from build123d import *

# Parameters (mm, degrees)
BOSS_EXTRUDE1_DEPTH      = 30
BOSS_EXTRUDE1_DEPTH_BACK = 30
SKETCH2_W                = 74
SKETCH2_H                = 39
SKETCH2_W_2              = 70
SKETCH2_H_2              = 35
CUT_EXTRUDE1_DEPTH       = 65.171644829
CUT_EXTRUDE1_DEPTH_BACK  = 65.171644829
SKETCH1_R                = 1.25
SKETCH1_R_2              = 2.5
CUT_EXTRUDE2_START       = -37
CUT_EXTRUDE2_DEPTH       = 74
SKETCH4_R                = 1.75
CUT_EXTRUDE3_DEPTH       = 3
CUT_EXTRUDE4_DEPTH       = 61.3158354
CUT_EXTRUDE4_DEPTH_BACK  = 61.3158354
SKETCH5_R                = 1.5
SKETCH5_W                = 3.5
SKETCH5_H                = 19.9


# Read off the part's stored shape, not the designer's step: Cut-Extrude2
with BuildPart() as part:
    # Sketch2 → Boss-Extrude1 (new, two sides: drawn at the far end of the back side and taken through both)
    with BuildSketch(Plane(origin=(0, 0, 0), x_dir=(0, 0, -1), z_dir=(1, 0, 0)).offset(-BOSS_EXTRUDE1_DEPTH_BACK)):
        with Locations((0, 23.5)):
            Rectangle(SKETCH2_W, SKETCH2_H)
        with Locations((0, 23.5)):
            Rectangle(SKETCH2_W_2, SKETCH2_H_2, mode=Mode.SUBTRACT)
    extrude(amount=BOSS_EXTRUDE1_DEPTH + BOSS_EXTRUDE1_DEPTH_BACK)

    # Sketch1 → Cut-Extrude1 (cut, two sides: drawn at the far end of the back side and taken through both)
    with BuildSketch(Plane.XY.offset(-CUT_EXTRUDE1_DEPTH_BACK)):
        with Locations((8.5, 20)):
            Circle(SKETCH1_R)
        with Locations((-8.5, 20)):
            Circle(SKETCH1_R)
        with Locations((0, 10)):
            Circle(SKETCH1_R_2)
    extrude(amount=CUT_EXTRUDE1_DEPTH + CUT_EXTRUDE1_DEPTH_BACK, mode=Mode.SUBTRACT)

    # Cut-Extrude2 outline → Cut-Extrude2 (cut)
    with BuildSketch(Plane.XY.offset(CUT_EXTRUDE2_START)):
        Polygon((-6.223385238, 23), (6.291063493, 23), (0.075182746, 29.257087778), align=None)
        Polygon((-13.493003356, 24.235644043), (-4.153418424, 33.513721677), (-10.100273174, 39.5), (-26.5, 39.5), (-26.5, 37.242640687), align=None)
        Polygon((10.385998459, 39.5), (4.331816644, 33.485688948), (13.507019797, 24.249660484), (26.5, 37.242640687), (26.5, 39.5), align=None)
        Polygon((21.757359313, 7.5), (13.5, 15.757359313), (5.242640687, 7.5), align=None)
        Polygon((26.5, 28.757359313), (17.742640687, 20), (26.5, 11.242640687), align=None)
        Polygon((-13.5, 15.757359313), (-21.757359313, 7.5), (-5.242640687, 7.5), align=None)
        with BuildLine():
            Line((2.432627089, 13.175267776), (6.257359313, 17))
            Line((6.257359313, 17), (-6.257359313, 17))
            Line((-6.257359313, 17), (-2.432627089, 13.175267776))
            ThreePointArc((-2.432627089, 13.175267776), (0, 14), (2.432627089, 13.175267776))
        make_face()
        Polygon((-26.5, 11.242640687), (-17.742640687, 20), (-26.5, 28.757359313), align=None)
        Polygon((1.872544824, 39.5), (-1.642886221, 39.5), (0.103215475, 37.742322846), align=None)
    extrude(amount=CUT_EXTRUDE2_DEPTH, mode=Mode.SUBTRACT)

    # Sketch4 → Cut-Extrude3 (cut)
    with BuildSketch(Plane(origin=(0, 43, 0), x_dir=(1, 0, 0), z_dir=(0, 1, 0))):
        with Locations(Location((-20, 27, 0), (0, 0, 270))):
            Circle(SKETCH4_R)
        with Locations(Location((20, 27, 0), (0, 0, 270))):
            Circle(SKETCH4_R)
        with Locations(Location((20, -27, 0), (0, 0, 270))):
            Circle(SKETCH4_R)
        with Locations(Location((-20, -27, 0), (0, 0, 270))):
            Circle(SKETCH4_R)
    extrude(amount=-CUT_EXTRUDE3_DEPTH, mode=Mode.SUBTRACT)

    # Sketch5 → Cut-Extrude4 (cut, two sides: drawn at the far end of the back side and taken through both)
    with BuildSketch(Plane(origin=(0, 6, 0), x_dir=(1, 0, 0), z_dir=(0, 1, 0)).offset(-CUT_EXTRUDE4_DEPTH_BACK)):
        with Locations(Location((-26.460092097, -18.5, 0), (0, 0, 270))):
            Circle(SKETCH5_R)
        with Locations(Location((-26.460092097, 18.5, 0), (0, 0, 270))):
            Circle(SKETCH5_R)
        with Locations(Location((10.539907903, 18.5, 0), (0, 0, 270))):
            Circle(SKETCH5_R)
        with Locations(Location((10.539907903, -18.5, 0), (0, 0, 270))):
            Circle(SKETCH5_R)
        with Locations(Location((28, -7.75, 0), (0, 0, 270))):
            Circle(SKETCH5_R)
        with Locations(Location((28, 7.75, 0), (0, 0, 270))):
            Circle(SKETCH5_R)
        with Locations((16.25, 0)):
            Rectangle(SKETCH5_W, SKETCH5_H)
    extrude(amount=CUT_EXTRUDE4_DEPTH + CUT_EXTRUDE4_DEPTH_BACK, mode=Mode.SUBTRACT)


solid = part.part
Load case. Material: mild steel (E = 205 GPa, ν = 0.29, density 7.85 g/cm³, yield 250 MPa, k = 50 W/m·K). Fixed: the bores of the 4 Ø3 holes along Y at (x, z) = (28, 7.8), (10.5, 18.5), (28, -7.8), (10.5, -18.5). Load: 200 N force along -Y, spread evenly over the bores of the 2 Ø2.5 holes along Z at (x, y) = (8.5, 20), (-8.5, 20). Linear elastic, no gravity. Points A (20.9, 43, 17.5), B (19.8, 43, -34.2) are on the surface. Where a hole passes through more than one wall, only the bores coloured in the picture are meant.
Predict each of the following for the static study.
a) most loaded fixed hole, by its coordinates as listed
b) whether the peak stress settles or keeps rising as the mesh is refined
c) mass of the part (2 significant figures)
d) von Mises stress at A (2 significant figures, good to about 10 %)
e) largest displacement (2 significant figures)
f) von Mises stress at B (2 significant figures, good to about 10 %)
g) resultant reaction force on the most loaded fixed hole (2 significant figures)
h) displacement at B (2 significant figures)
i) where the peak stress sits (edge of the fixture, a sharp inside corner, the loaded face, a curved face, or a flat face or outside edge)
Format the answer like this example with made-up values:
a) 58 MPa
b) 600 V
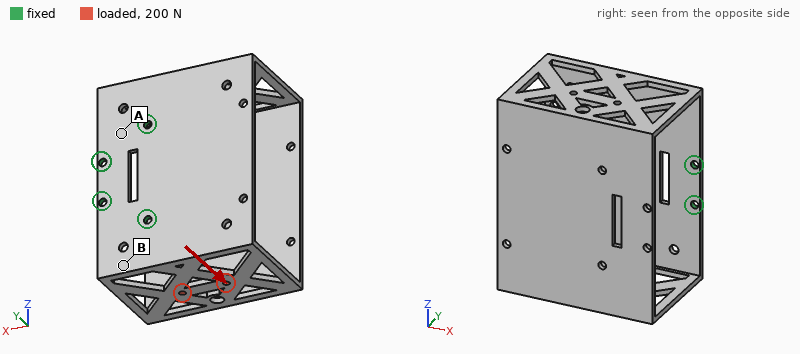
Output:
a) (10.5, -18.5)
b) keeps rising
c) 180 g
d) 18 MPa
e) 0.18 mm
f) 33 MPa
g) 280 N
h) 0.040 mm
i) edge of the fixture
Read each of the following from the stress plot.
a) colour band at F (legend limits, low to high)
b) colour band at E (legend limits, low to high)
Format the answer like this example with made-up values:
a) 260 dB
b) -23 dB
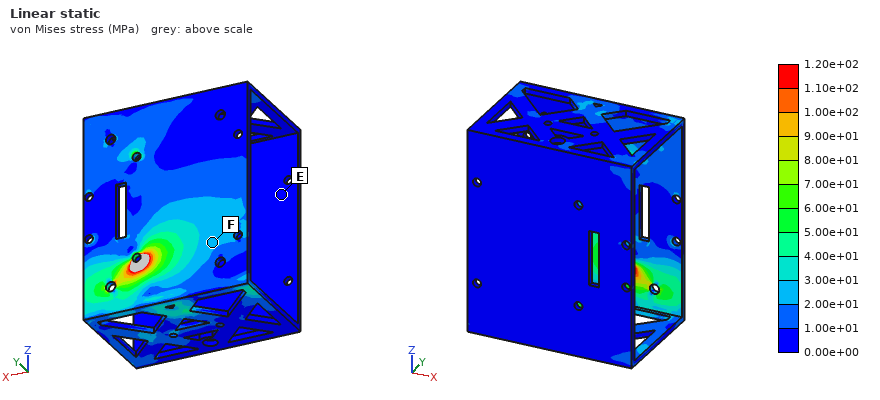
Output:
a) 2.00e+01 to 3.00e+01 MPa
b) 0.00e+00 to 1.00e+01 MPa
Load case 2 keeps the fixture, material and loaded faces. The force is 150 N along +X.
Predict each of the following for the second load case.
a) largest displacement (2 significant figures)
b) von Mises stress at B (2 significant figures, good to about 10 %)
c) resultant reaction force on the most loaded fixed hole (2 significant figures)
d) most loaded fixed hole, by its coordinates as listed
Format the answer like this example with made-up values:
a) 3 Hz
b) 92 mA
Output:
a) 0.20 mm
b) 28 MPa
c) 180 N
d) (10.5, -18.5)
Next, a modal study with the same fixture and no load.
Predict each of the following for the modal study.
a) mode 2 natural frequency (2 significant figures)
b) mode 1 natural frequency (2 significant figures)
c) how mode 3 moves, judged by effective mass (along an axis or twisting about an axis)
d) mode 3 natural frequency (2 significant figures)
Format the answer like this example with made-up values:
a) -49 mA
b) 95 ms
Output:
a) 420 Hz
b) 420 Hz
c) twisting about Y
d) 900 Hz
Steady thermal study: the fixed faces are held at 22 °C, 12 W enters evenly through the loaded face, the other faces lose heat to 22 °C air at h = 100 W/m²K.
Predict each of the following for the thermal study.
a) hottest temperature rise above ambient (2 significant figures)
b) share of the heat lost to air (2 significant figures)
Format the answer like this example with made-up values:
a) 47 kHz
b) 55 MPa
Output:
a) 54 K
b) 94 %
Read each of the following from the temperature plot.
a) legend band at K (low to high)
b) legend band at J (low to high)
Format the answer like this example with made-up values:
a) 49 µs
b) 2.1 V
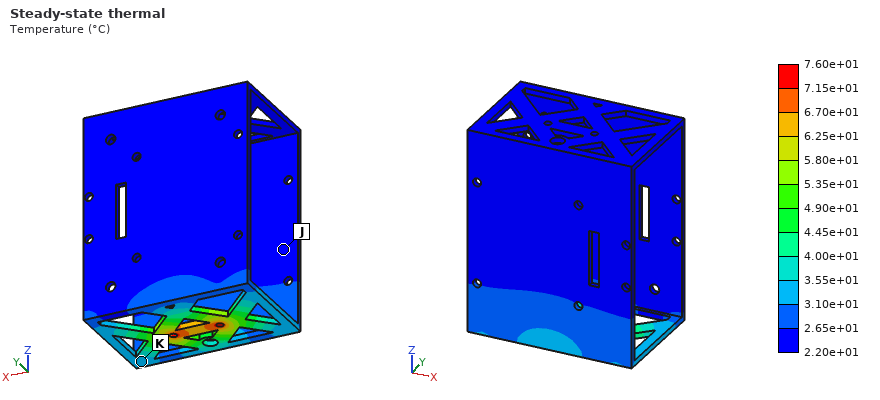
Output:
a) 3.10e+01 to 3.55e+01 °C
b) 2.20e+01 to 2.65e+01 °C
